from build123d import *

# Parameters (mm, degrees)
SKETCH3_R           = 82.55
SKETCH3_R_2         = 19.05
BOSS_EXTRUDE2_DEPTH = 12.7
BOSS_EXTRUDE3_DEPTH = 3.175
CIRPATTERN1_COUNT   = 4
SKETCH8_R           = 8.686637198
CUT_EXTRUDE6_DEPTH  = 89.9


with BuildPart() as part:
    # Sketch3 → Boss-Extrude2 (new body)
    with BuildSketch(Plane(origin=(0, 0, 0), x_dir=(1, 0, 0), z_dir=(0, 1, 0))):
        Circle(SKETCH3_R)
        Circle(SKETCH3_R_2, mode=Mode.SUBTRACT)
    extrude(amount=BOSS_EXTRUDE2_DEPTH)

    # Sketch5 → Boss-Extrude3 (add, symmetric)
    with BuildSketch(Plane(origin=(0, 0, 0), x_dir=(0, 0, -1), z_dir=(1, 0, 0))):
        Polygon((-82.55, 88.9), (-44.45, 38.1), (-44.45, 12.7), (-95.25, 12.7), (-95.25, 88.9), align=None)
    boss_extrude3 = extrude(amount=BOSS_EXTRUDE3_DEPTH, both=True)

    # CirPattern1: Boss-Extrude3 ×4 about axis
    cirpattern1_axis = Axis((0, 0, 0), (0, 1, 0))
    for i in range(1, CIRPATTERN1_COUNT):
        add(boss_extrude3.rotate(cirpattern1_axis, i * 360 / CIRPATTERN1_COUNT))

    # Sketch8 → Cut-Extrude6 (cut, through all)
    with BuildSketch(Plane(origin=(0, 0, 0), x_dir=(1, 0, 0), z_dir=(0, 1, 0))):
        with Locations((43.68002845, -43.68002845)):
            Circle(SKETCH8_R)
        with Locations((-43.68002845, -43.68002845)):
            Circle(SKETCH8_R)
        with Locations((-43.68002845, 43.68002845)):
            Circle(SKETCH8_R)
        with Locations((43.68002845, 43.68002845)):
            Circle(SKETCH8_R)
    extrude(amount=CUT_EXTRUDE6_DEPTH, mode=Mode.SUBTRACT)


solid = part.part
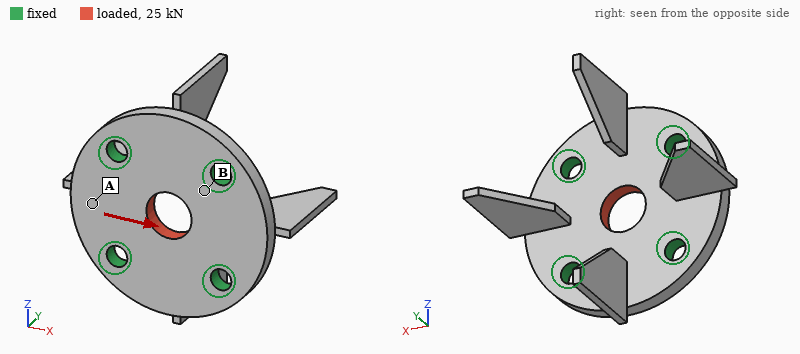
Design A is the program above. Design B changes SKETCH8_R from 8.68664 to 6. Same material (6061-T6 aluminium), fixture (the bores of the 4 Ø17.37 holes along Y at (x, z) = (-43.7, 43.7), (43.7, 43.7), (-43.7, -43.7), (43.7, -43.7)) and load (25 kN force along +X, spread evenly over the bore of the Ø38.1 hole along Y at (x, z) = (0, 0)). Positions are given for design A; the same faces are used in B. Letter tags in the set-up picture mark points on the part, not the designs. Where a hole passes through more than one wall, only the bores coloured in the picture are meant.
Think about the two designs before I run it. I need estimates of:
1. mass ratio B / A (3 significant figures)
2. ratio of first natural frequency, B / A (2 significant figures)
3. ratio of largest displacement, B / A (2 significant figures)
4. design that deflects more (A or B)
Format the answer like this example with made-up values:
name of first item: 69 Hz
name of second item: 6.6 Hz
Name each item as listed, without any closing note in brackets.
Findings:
mass ratio B / A: 1.02
ratio of first natural frequency, B / A: 1.0
ratio of largest displacement, B / A: 1.1
design that deflects more: B
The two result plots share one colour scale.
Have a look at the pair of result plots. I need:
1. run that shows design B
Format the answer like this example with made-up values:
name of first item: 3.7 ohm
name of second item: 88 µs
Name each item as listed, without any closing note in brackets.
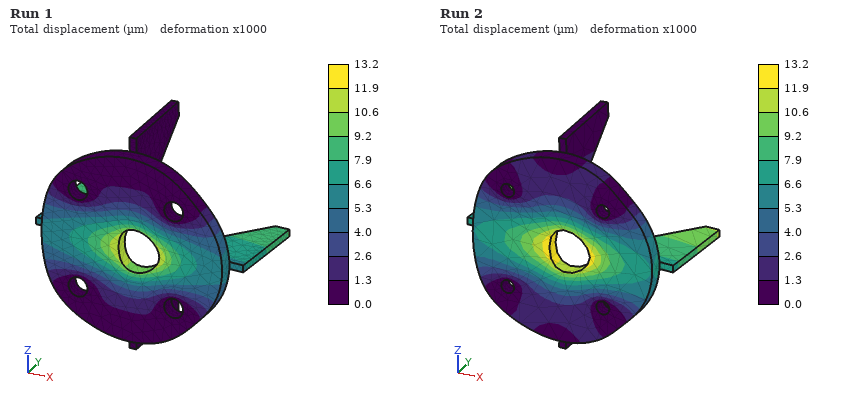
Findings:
run that shows design B: Run 2
